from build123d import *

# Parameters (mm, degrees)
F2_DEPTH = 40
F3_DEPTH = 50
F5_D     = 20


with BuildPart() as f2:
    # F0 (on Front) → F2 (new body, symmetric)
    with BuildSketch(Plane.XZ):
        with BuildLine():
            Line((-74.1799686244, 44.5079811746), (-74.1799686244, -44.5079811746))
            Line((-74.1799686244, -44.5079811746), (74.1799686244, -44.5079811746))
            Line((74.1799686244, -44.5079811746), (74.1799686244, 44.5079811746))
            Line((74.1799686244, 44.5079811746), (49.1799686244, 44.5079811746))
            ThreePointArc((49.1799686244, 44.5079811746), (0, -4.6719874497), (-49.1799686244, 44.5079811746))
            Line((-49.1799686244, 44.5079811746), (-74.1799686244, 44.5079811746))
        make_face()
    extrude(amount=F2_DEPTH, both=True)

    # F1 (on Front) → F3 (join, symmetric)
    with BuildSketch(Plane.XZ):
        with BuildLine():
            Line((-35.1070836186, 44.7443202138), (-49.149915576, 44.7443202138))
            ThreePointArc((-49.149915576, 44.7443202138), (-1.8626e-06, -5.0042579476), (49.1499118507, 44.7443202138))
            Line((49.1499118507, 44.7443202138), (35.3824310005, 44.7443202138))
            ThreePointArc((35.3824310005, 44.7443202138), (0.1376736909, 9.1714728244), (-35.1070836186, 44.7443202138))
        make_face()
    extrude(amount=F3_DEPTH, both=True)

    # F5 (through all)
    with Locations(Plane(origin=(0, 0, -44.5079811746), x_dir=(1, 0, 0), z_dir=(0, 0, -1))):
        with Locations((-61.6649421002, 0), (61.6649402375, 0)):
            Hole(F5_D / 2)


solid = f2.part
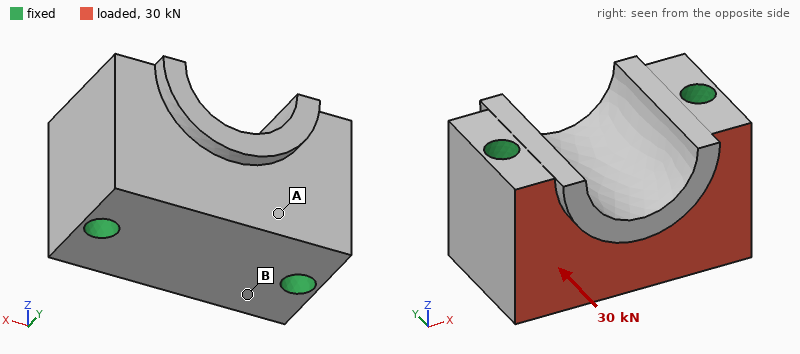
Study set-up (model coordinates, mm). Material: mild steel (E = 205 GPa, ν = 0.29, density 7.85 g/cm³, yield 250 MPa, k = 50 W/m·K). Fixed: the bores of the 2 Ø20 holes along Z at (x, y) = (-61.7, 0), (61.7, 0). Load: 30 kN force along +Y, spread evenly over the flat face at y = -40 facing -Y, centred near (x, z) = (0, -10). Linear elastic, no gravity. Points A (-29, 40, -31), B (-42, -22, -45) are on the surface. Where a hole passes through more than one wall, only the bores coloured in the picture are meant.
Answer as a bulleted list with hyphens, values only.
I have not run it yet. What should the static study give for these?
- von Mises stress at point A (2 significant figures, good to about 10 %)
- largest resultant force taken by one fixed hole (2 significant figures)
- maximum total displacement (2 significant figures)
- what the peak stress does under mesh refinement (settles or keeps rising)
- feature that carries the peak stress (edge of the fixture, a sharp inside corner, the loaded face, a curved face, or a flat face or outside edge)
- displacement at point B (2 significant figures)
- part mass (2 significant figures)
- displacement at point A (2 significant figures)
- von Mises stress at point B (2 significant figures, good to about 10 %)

- 2.0 MPa
- 15 kN
- 2.0 µm
- keeps rising
- edge of the fixture
- 0.96 µm
- 6.9 kg
- 0.90 µm
- 4.5 MPa
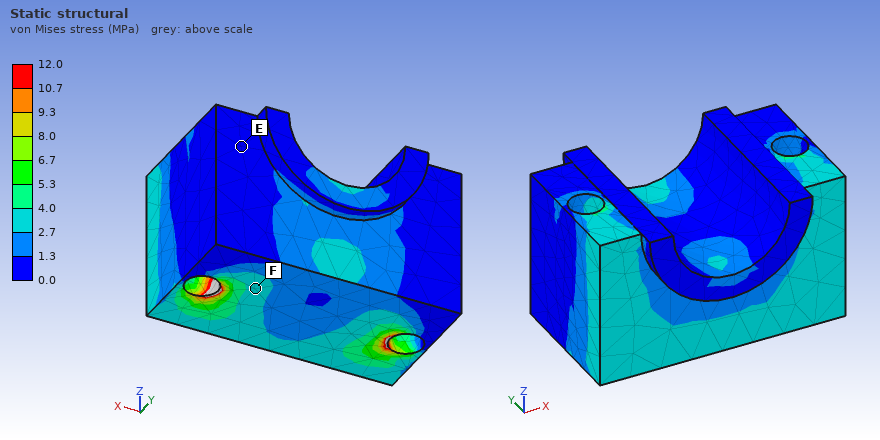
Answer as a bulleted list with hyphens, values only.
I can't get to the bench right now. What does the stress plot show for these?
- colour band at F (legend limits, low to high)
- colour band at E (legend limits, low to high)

- 2.7 to 4.0 MPa
- 0.0 to 1.3 MPa
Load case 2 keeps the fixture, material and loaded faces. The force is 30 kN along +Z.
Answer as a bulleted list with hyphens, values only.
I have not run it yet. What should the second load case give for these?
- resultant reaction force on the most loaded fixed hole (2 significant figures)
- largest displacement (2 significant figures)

- 15 kN
- 4.3 µm
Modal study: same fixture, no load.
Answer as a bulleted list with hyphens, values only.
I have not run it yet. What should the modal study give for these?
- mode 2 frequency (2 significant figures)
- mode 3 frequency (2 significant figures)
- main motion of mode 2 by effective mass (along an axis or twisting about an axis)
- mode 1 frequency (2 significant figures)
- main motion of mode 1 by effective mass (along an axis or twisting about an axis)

- 11 kHz
- 13 kHz
- along Z
- 9800 Hz
- along Y
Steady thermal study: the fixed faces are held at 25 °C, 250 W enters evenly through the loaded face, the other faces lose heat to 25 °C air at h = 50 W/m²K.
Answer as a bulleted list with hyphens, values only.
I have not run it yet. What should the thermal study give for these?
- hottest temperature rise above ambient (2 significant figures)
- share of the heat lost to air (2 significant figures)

- 24 K
- 7.0 %
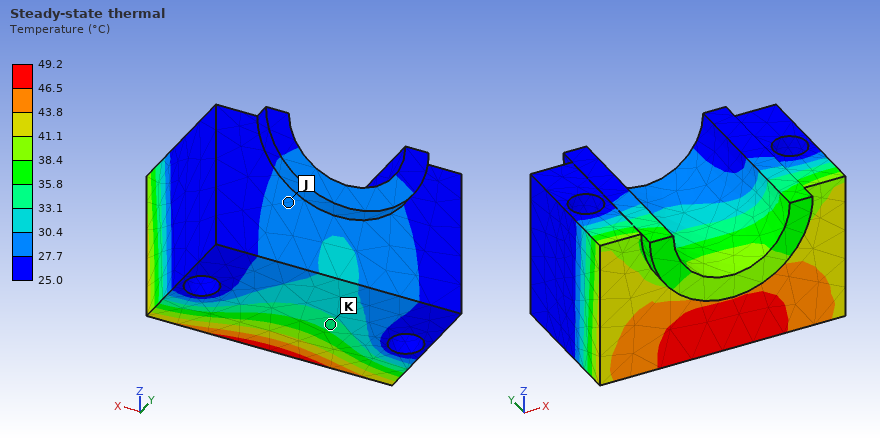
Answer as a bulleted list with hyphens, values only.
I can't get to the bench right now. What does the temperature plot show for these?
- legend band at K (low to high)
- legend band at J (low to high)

- 33.1 to 35.8 °C
- 27.7 to 30.4 °C
